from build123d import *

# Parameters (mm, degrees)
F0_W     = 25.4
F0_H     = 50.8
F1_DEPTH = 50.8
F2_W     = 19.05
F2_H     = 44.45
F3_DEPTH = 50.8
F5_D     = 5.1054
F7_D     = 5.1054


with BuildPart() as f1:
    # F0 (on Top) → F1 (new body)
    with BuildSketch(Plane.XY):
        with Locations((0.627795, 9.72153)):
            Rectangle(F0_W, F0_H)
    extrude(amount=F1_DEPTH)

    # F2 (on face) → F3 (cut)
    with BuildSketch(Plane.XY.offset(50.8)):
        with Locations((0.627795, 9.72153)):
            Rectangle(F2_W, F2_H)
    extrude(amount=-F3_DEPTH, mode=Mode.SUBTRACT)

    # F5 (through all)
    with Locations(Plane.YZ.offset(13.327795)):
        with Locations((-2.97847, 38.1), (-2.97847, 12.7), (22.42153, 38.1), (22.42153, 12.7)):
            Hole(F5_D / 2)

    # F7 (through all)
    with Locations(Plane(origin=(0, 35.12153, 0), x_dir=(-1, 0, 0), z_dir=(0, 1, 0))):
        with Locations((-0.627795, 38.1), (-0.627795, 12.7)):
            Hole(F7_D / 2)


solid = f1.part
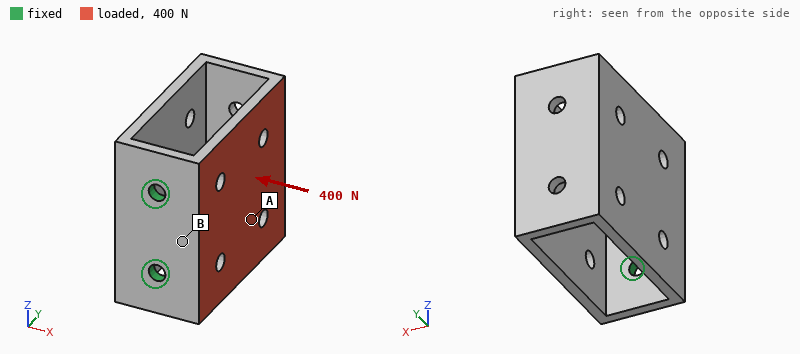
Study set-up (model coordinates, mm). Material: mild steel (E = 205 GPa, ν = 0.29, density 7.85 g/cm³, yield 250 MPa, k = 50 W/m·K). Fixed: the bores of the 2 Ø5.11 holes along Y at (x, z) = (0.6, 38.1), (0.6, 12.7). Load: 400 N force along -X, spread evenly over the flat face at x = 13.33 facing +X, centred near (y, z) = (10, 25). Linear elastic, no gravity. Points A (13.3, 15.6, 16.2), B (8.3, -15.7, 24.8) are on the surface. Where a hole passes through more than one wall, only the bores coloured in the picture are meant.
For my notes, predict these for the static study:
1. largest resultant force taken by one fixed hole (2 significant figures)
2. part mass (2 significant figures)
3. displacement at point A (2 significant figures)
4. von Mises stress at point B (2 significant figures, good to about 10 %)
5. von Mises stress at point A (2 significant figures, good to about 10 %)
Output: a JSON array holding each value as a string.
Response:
["200 N", "170 g", "67 µm", "39 MPa", "15 MPa"]
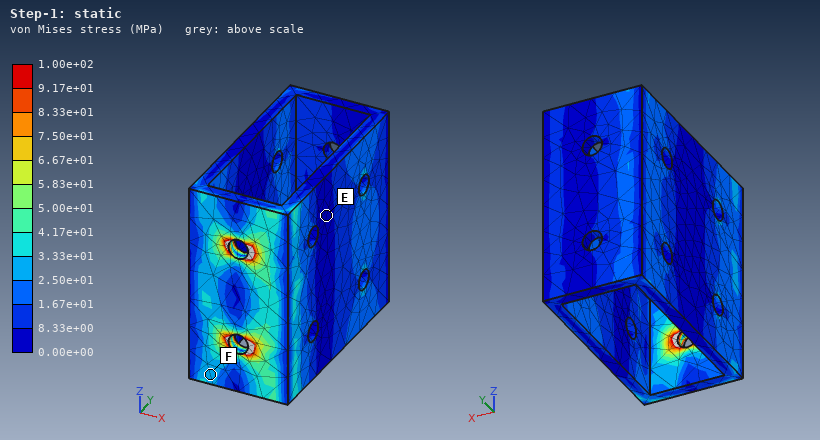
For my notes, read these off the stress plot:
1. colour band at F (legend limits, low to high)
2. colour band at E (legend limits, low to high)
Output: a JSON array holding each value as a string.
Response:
["2.50e+01 to 3.33e+01 MPa", "0.00e+00 to 8.33e+00 MPa"]
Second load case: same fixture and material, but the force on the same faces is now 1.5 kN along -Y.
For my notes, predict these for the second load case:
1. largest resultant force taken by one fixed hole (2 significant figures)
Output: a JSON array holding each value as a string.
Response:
["750 N"]
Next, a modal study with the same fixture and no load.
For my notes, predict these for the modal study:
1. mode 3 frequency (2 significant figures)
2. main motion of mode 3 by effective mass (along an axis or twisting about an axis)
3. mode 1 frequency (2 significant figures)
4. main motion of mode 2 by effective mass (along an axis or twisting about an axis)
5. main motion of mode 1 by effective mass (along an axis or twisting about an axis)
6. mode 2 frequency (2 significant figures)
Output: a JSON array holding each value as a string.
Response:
["3000 Hz", "twisting about Y", "890 Hz", "along Z", "along X", "2500 Hz"]
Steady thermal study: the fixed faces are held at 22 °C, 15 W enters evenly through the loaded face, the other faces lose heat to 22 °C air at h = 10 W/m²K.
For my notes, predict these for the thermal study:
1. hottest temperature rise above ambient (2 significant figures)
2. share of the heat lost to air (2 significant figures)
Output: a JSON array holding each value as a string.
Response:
["37 K", "17 %"]
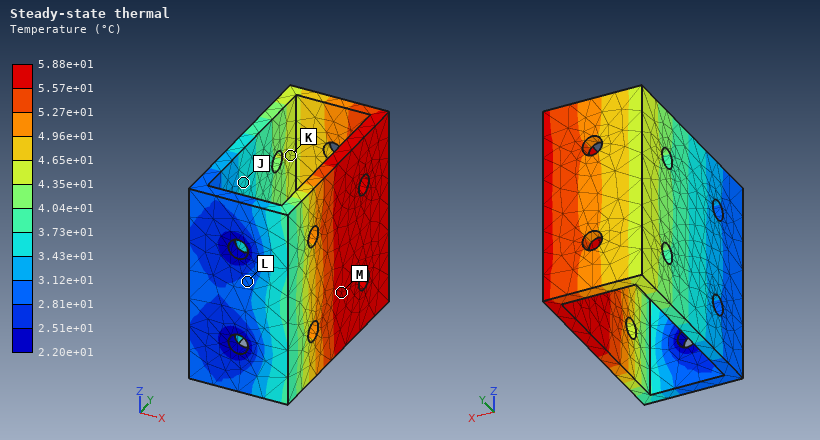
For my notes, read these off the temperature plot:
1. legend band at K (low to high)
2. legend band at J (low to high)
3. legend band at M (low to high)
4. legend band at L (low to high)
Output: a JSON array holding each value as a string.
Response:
["4.35e+01 to 4.65e+01 °C", "3.43e+01 to 3.73e+01 °C", "5.57e+01 to 5.88e+01 °C", "2.81e+01 to 3.12e+01 °C"]
